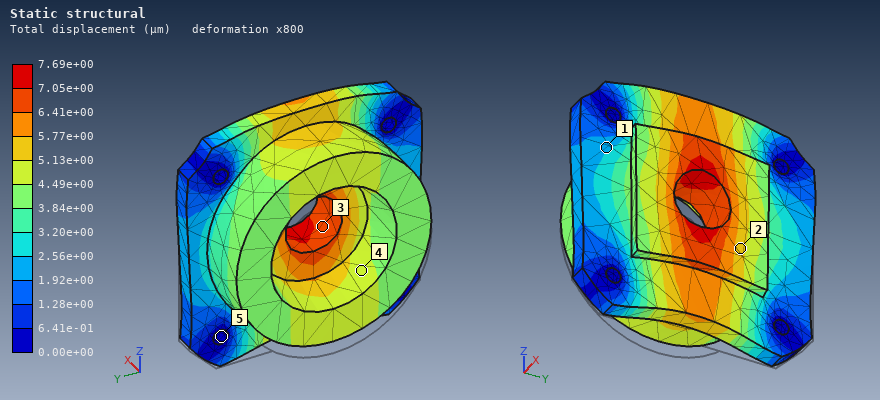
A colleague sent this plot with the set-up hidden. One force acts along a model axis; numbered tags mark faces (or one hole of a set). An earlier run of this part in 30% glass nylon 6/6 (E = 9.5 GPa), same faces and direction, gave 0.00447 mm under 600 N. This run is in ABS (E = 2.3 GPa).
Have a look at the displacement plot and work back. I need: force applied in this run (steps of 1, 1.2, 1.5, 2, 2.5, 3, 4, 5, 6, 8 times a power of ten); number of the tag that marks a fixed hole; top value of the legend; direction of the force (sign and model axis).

250 N
5
7.69e+00 µm
+Z
